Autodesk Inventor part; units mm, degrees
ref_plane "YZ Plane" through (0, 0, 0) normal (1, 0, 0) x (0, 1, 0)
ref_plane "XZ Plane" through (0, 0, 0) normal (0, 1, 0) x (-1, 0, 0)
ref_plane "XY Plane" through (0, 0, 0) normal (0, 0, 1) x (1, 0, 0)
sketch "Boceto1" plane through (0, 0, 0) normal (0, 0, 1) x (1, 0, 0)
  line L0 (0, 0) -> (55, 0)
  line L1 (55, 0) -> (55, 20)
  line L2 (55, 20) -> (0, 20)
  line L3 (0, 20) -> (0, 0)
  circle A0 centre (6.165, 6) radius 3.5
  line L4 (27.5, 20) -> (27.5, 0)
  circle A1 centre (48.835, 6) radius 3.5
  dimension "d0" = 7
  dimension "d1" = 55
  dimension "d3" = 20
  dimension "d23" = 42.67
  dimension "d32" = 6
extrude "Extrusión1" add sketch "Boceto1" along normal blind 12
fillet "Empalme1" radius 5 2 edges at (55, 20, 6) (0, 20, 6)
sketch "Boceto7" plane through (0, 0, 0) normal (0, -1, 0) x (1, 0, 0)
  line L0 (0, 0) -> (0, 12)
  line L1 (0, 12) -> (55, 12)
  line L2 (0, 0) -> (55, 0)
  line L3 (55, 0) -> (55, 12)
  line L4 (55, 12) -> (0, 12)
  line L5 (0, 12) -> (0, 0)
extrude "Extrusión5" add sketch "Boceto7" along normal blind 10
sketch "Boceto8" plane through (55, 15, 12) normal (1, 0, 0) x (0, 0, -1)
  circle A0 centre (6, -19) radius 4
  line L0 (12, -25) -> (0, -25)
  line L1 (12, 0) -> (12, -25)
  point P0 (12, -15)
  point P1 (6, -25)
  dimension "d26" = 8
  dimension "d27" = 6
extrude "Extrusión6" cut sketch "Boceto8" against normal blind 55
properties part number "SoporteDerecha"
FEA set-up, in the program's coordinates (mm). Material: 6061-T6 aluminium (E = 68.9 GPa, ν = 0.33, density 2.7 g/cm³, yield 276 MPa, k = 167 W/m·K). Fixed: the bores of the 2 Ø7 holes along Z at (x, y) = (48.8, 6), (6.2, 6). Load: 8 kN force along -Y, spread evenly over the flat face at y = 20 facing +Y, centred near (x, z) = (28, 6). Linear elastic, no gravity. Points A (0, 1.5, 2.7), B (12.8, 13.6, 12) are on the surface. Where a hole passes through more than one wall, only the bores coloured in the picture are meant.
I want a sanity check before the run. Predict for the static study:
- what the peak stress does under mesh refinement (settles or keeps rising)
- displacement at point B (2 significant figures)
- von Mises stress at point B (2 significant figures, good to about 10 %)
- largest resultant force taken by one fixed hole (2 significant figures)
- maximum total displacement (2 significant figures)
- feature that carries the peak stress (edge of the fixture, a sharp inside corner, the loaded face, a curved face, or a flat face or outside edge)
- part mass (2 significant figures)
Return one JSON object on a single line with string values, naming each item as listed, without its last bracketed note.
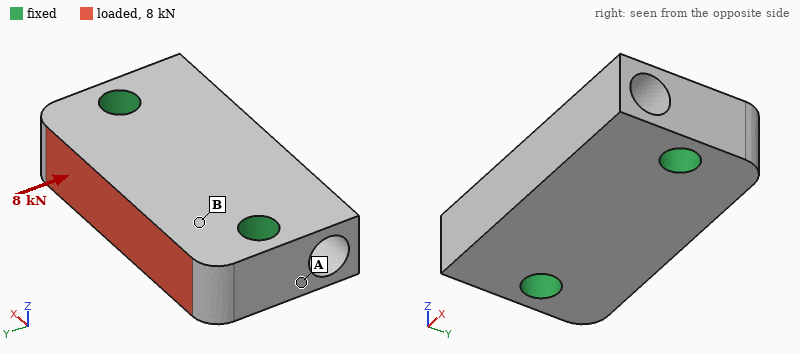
{"what the peak stress does under mesh refinement": "keeps rising", "displacement at point B": "4.4 µm", "von Mises stress at point B": "21 MPa", "largest resultant force taken by one fixed hole": "4.1 kN", "maximum total displacement": "9.6 µm", "feature that carries the peak stress": "edge of the fixture", "part mass": "43 g"}
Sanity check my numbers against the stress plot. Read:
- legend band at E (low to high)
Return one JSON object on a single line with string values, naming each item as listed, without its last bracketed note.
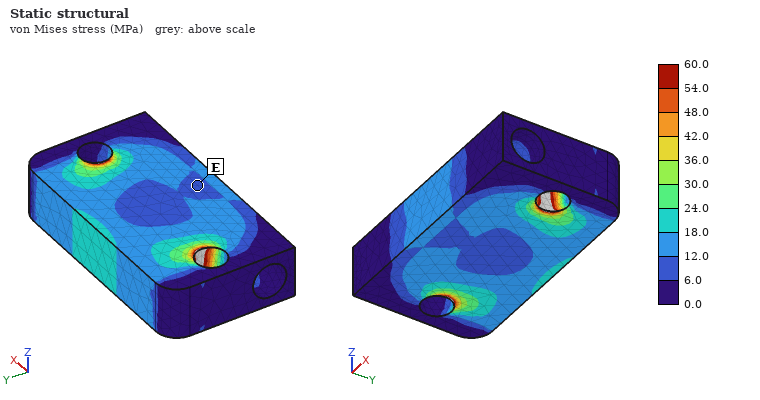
{"legend band at E": "6.0 to 12.0 MPa"}
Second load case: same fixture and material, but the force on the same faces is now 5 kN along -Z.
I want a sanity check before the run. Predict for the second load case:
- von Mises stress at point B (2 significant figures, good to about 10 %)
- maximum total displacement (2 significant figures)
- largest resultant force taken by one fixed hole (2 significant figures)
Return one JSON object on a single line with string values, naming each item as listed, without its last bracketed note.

{"von Mises stress at point B": "40 MPa", "maximum total displacement": "33 µm", "largest resultant force taken by one fixed hole": "2.5 kN"}
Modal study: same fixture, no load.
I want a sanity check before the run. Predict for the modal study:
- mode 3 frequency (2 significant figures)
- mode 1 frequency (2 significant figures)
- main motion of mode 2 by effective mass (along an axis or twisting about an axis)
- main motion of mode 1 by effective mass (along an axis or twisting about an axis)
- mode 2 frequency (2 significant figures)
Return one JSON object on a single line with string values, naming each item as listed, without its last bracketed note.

{"mode 3 frequency": "27 kHz", "mode 1 frequency": "19 kHz", "main motion of mode 2 by effective mass": "along Z", "main motion of mode 1 by effective mass": "along Z", "mode 2 frequency": "23 kHz"}
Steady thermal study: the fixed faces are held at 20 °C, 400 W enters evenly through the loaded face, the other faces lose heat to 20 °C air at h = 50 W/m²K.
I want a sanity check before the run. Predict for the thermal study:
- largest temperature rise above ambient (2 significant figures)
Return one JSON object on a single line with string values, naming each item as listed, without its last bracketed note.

{"largest temperature rise above ambient": "83 K"}
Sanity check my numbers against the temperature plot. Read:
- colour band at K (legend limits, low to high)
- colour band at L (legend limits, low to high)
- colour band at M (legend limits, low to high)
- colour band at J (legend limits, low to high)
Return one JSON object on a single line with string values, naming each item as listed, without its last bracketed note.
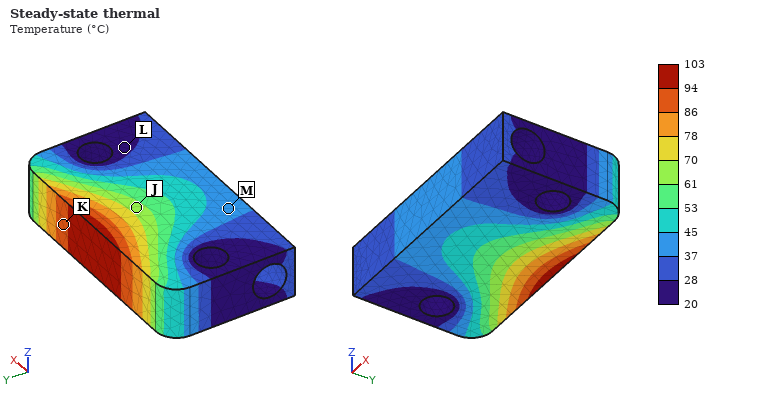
{"colour band at K": "86 to 94 °C", "colour band at L": "20 to 28 °C", "colour band at M": "37 to 45 °C", "colour band at J": "61 to 70 °C"}
